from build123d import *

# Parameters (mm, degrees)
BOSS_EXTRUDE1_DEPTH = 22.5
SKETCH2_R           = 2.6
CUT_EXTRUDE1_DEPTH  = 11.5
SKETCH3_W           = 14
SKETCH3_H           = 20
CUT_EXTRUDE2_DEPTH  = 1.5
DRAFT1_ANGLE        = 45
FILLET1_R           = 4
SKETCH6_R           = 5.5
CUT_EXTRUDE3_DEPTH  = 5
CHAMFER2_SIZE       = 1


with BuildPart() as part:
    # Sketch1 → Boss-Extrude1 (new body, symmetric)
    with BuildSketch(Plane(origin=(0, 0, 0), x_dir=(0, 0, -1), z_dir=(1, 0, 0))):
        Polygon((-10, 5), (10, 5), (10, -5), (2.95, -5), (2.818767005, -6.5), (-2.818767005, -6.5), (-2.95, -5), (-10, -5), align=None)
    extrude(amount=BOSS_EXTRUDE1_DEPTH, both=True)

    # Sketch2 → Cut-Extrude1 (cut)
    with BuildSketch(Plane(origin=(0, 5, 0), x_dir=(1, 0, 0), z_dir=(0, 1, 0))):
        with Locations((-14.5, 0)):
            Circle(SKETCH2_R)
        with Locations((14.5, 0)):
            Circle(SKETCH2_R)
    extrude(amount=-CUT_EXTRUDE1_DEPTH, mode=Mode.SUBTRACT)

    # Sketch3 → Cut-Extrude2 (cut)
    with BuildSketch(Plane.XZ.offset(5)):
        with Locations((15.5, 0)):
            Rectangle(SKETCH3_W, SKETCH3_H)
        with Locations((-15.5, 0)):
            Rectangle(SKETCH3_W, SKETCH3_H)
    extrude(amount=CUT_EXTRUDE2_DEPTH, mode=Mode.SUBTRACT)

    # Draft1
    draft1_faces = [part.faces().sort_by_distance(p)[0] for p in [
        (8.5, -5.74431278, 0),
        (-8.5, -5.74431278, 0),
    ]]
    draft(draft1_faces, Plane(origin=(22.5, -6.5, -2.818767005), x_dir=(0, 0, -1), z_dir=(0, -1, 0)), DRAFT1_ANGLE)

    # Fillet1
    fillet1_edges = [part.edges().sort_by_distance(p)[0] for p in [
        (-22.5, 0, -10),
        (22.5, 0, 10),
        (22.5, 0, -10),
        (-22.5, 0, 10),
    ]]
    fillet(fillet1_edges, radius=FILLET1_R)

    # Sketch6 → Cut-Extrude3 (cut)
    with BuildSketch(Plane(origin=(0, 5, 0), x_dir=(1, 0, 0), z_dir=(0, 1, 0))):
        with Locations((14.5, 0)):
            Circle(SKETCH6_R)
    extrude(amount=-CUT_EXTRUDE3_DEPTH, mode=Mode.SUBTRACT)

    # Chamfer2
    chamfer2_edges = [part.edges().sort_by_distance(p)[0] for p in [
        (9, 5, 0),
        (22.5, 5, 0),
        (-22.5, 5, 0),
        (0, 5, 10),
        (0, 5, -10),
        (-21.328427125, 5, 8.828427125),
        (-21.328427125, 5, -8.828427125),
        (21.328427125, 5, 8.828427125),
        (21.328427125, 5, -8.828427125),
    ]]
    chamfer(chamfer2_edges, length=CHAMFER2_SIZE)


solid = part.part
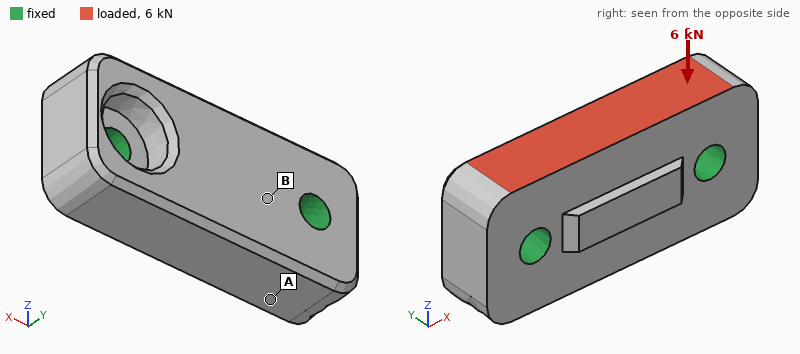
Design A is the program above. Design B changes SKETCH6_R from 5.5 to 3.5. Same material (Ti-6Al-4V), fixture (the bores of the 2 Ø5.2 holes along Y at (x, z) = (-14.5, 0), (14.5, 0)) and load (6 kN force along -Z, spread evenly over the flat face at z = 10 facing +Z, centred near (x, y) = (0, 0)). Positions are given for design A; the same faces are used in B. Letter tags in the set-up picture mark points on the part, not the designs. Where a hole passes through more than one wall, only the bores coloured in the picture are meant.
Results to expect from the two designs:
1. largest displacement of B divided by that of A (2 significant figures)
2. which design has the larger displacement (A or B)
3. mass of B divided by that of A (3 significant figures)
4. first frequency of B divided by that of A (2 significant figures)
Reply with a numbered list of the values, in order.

1. 0.79
2. A
3. 1.04
4. 1.0
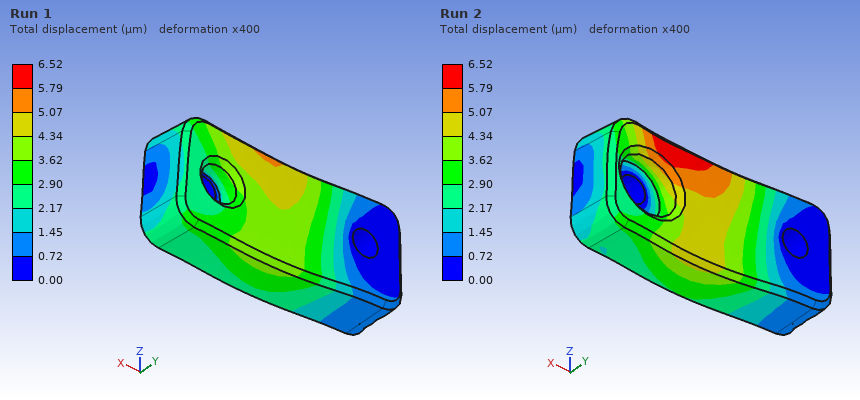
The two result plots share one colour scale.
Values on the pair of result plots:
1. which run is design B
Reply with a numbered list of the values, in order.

1. Run 1
